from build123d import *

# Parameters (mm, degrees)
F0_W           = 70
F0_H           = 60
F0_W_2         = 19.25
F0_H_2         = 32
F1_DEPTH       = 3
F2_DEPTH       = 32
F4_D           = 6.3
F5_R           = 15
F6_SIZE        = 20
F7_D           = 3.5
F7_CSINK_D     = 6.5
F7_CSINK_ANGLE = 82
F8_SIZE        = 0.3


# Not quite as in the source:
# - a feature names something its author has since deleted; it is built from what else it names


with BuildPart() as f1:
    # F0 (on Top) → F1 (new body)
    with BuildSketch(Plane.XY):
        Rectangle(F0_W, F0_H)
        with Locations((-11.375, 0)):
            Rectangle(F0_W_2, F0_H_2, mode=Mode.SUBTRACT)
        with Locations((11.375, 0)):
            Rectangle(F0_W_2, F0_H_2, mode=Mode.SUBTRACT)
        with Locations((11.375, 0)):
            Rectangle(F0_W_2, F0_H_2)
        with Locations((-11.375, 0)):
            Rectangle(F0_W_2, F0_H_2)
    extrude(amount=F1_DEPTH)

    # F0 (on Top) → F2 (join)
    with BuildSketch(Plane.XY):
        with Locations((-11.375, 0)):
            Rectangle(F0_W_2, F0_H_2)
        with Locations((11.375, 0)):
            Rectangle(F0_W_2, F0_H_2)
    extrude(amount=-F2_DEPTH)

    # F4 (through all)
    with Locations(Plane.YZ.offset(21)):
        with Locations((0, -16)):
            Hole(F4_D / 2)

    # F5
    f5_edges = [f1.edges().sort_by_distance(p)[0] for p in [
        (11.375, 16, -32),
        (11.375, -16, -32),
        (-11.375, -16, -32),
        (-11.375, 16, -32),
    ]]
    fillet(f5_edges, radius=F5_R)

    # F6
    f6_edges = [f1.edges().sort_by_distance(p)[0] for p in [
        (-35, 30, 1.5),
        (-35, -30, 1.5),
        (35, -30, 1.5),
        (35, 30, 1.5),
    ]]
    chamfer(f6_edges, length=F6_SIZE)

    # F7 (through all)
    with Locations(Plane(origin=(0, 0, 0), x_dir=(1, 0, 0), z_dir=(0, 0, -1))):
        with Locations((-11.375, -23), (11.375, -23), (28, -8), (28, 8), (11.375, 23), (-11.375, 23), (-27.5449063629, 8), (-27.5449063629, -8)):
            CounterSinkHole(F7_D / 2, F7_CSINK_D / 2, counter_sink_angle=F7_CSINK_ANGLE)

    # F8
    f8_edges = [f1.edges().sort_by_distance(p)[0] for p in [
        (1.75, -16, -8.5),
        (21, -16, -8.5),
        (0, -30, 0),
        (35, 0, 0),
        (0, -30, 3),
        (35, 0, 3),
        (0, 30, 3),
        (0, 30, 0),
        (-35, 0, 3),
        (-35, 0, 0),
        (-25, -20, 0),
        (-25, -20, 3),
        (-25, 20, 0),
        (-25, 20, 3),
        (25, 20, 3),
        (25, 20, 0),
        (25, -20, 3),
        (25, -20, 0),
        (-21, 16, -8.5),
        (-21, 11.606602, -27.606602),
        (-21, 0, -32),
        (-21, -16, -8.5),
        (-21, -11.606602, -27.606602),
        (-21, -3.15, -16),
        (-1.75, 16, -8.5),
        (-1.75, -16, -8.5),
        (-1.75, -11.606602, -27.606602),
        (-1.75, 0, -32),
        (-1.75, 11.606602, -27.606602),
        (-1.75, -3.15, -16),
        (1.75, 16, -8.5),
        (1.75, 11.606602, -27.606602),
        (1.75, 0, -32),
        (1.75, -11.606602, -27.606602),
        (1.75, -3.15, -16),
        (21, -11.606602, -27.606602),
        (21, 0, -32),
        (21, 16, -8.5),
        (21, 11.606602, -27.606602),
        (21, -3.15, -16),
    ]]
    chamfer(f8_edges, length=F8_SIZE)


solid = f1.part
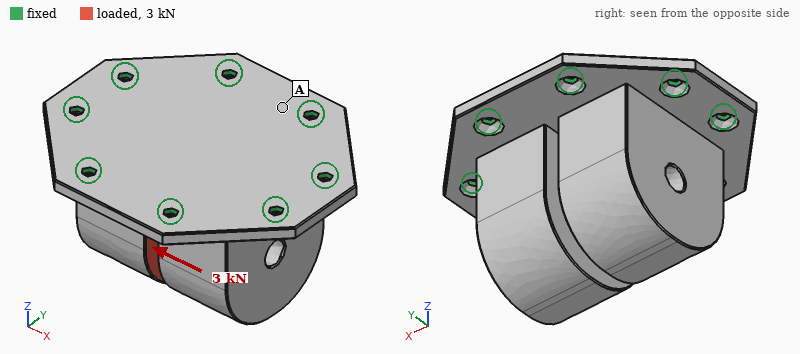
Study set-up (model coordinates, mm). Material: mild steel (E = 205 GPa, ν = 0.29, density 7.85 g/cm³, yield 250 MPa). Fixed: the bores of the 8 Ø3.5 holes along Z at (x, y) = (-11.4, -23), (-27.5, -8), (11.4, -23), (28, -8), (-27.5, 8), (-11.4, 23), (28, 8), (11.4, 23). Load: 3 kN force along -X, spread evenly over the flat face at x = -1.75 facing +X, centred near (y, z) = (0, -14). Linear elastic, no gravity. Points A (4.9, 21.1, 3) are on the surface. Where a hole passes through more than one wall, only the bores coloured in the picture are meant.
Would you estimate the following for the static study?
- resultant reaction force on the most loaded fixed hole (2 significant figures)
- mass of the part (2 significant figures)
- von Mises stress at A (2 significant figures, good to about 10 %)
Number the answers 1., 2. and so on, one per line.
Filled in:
1. 1.4 kN
2. 350 g
3. 27 MPa
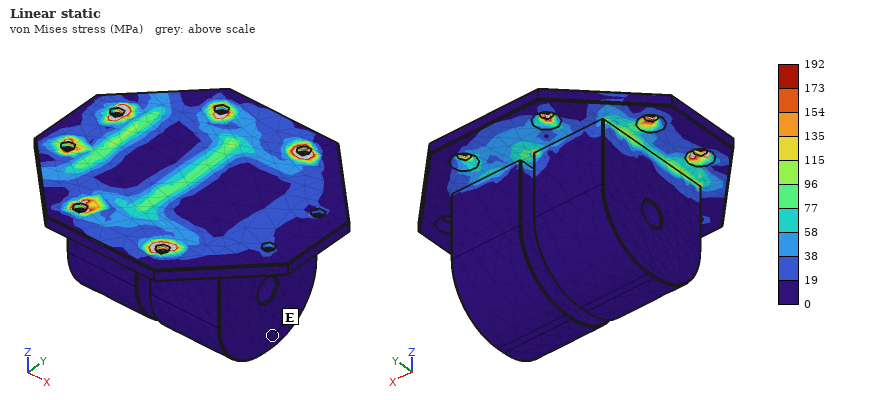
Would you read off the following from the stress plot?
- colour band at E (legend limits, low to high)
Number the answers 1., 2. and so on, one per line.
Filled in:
1. 0 to 19 MPa
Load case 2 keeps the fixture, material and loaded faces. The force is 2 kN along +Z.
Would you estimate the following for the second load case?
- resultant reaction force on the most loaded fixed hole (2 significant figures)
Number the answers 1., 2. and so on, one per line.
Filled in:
1. 920 N
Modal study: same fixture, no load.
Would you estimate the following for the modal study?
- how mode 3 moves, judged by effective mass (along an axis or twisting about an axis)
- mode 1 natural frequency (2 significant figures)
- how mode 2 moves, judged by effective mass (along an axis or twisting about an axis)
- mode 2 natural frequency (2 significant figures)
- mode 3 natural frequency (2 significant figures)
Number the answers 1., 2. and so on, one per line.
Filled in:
1. along X
2. 3300 Hz
3. along Y
4. 5900 Hz
5. 6200 Hz
